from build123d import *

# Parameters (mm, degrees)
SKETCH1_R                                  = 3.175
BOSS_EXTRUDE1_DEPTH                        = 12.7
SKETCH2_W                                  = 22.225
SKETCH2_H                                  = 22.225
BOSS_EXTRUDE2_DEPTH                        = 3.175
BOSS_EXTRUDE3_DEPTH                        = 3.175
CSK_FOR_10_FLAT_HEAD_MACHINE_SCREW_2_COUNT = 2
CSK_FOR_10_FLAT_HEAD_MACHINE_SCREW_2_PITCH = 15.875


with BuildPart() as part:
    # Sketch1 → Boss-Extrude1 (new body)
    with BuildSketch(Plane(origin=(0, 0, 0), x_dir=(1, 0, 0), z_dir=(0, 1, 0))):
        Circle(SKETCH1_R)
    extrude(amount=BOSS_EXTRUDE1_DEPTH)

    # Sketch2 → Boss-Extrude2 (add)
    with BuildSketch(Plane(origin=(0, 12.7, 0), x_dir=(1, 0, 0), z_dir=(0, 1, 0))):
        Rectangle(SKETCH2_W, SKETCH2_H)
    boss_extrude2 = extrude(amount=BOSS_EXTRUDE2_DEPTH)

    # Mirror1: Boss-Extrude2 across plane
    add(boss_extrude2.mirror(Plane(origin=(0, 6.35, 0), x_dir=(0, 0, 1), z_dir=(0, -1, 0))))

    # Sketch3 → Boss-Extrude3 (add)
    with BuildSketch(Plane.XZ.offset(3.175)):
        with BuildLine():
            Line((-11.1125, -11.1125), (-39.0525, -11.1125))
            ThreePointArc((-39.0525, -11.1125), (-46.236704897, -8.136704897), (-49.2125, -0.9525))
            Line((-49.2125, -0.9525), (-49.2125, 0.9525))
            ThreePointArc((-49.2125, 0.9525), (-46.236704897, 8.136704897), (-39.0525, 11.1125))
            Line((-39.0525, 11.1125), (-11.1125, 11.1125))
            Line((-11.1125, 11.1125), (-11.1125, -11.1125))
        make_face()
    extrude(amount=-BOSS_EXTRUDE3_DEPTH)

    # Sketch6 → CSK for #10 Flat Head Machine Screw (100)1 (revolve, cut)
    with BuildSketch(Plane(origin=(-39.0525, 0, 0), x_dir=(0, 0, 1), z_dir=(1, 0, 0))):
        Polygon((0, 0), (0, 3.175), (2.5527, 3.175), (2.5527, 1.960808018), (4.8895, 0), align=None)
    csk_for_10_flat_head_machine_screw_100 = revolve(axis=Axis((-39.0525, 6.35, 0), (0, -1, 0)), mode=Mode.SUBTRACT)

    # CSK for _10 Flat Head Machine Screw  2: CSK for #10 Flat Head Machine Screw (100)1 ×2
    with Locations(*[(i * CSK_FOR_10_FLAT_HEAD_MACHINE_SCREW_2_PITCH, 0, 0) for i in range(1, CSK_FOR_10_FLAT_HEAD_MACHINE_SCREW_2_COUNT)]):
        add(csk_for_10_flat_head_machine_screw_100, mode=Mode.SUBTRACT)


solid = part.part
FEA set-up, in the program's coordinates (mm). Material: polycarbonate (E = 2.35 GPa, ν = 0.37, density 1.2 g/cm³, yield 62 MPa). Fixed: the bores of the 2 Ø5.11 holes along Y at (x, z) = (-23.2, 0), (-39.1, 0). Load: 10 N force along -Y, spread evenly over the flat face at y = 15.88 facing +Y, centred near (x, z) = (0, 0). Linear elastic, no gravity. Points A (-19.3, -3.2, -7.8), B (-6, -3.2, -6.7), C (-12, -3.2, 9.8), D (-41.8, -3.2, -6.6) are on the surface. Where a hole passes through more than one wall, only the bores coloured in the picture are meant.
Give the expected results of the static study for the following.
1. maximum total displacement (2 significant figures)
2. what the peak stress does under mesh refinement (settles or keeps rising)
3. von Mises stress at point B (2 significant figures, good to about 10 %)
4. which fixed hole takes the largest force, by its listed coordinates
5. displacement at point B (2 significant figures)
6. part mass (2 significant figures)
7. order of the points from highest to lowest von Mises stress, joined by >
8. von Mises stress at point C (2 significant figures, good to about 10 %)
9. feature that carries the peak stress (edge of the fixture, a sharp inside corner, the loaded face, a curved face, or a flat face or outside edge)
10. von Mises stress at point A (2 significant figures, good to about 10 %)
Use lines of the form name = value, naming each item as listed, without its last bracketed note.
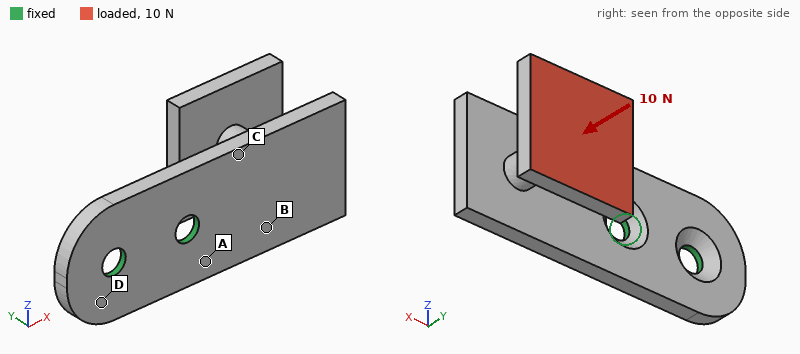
maximum total displacement = 0.77 mm
what the peak stress does under mesh refinement = keeps rising
von Mises stress at point B = 1.6 MPa
which fixed hole takes the largest force, by its listed coordinates = (-23.2, 0)
displacement at point B = 0.25 mm
part mass = 7.0 g
order of the points from highest to lowest von Mises stress, joined by > = A > C > B > D
von Mises stress at point C = 3.1 MPa
feature that carries the peak stress = edge of the fixture
von Mises stress at point A = 4.5 MPa
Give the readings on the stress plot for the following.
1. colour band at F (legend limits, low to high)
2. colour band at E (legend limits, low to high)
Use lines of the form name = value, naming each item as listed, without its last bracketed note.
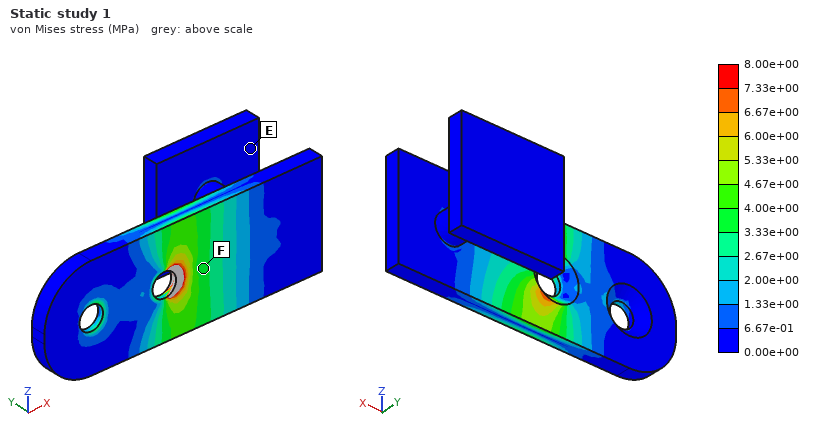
colour band at F = 3.33e+00 to 4.00e+00 MPa
colour band at E = 0.00e+00 to 6.67e-01 MPa
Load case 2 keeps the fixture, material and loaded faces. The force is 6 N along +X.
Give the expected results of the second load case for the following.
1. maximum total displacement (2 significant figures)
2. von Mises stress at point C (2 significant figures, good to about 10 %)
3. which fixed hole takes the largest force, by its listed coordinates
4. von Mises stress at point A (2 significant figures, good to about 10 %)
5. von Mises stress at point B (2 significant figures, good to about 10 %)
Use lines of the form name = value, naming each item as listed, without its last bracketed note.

maximum total displacement = 0.63 mm
von Mises stress at point C = 2.7 MPa
which fixed hole takes the largest force, by its listed coordinates = (-39.1, 0)
von Mises stress at point A = 2.5 MPa
von Mises stress at point B = 2.5 MPa
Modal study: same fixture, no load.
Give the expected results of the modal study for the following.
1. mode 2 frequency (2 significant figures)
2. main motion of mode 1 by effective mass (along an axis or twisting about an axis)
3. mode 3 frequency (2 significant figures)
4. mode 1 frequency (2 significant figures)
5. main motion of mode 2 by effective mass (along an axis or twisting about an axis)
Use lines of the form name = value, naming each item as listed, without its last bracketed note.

mode 2 frequency = 470 Hz
main motion of mode 1 by effective mass = along Y
mode 3 frequency = 980 Hz
mode 1 frequency = 300 Hz
main motion of mode 2 by effective mass = along Z
